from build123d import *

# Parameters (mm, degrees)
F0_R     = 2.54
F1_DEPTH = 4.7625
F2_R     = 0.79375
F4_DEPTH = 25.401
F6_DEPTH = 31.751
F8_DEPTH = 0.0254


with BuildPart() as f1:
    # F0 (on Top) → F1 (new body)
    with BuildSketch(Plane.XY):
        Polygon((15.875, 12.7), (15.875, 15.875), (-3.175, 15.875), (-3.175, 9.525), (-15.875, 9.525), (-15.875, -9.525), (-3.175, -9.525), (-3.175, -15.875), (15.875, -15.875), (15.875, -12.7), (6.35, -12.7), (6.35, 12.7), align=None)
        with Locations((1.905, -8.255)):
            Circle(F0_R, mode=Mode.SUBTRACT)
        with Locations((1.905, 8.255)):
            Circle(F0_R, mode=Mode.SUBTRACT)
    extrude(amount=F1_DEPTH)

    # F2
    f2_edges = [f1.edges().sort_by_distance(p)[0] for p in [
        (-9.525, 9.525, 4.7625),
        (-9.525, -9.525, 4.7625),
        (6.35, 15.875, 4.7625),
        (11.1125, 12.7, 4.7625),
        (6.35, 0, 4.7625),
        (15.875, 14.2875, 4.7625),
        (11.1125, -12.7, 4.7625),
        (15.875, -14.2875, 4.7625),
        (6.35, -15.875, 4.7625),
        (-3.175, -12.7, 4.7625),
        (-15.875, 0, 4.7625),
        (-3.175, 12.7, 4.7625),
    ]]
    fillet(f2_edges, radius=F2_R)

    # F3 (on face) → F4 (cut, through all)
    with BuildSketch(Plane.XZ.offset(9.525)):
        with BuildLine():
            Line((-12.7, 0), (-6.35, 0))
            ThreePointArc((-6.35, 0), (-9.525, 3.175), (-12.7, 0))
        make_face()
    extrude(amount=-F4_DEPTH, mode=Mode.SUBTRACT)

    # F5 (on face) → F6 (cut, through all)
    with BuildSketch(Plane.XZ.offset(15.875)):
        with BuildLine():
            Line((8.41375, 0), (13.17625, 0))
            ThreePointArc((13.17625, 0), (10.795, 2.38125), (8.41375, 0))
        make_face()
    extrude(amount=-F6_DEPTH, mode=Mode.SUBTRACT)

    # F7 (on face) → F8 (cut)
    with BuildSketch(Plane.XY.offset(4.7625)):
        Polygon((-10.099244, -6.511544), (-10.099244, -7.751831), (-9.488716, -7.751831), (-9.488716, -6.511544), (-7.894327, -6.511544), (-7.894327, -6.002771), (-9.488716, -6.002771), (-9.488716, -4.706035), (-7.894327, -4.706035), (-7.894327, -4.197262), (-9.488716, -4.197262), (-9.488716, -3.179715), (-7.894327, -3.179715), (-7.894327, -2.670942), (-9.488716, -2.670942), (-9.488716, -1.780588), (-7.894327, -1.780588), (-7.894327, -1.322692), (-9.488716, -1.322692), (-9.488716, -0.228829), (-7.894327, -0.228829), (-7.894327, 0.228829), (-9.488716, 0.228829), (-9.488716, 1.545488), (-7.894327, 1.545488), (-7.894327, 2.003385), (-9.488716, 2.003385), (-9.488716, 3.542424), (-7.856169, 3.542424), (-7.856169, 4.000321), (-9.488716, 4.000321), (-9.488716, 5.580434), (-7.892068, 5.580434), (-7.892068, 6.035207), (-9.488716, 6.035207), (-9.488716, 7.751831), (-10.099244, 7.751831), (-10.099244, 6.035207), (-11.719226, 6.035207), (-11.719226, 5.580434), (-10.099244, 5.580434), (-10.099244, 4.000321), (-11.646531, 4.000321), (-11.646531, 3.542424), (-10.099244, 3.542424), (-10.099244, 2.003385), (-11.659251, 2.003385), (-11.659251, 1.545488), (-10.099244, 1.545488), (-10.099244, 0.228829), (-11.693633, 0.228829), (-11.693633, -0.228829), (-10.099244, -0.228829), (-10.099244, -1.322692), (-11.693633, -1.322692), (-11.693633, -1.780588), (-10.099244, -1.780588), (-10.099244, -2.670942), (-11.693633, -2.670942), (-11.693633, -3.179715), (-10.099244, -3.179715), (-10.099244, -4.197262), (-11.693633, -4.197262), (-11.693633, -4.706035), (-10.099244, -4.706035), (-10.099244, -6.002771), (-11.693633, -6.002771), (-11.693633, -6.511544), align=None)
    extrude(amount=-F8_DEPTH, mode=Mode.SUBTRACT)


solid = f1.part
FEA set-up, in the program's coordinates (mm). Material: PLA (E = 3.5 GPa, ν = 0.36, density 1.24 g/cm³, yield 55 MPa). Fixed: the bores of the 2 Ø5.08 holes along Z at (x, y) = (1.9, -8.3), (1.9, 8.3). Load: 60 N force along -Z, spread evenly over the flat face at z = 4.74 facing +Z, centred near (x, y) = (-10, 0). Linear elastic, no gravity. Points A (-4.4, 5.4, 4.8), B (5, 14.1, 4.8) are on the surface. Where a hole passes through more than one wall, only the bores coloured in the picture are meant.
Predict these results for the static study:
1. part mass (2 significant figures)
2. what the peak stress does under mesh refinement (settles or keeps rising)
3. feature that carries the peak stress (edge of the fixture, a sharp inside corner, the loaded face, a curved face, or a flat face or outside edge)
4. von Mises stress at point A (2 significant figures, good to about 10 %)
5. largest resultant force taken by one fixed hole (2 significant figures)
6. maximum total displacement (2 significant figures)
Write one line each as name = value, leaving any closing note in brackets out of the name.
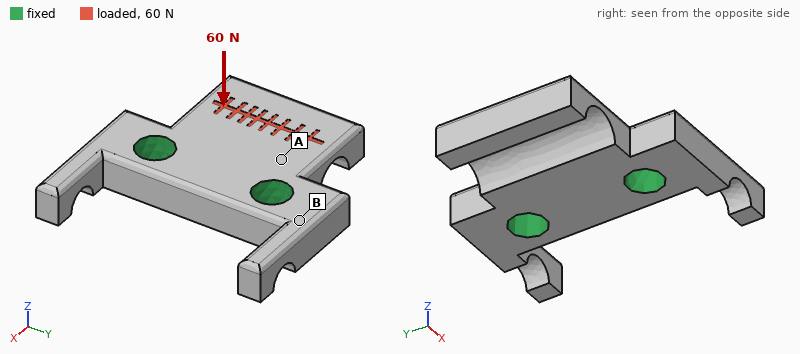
part mass = 2.9 g
what the peak stress does under mesh refinement = keeps rising
feature that carries the peak stress = a sharp inside corner
von Mises stress at point A = 5.3 MPa
largest resultant force taken by one fixed hole = 32 N
maximum total displacement = 0.15 mm
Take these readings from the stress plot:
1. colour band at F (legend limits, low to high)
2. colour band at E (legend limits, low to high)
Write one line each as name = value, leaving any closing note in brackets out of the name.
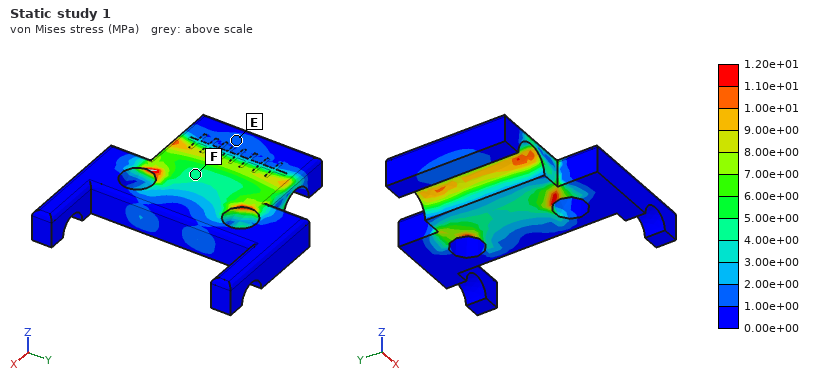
colour band at F = 4.00e+00 to 5.00e+00 MPa
colour band at E = 1.00e+00 to 2.00e+00 MPa
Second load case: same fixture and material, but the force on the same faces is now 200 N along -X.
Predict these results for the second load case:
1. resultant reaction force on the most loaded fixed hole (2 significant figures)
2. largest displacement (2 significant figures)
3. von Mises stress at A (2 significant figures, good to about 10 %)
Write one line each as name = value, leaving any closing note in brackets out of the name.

resultant reaction force on the most loaded fixed hole = 110 N
largest displacement = 0.21 mm
von Mises stress at A = 9.4 MPa
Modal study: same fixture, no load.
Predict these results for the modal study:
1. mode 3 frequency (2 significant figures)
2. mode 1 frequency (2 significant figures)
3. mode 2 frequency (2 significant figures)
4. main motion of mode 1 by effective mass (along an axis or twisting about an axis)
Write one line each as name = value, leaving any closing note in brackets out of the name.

mode 3 frequency = 5800 Hz
mode 1 frequency = 3100 Hz
mode 2 frequency = 5800 Hz
main motion of mode 1 by effective mass = along Z
